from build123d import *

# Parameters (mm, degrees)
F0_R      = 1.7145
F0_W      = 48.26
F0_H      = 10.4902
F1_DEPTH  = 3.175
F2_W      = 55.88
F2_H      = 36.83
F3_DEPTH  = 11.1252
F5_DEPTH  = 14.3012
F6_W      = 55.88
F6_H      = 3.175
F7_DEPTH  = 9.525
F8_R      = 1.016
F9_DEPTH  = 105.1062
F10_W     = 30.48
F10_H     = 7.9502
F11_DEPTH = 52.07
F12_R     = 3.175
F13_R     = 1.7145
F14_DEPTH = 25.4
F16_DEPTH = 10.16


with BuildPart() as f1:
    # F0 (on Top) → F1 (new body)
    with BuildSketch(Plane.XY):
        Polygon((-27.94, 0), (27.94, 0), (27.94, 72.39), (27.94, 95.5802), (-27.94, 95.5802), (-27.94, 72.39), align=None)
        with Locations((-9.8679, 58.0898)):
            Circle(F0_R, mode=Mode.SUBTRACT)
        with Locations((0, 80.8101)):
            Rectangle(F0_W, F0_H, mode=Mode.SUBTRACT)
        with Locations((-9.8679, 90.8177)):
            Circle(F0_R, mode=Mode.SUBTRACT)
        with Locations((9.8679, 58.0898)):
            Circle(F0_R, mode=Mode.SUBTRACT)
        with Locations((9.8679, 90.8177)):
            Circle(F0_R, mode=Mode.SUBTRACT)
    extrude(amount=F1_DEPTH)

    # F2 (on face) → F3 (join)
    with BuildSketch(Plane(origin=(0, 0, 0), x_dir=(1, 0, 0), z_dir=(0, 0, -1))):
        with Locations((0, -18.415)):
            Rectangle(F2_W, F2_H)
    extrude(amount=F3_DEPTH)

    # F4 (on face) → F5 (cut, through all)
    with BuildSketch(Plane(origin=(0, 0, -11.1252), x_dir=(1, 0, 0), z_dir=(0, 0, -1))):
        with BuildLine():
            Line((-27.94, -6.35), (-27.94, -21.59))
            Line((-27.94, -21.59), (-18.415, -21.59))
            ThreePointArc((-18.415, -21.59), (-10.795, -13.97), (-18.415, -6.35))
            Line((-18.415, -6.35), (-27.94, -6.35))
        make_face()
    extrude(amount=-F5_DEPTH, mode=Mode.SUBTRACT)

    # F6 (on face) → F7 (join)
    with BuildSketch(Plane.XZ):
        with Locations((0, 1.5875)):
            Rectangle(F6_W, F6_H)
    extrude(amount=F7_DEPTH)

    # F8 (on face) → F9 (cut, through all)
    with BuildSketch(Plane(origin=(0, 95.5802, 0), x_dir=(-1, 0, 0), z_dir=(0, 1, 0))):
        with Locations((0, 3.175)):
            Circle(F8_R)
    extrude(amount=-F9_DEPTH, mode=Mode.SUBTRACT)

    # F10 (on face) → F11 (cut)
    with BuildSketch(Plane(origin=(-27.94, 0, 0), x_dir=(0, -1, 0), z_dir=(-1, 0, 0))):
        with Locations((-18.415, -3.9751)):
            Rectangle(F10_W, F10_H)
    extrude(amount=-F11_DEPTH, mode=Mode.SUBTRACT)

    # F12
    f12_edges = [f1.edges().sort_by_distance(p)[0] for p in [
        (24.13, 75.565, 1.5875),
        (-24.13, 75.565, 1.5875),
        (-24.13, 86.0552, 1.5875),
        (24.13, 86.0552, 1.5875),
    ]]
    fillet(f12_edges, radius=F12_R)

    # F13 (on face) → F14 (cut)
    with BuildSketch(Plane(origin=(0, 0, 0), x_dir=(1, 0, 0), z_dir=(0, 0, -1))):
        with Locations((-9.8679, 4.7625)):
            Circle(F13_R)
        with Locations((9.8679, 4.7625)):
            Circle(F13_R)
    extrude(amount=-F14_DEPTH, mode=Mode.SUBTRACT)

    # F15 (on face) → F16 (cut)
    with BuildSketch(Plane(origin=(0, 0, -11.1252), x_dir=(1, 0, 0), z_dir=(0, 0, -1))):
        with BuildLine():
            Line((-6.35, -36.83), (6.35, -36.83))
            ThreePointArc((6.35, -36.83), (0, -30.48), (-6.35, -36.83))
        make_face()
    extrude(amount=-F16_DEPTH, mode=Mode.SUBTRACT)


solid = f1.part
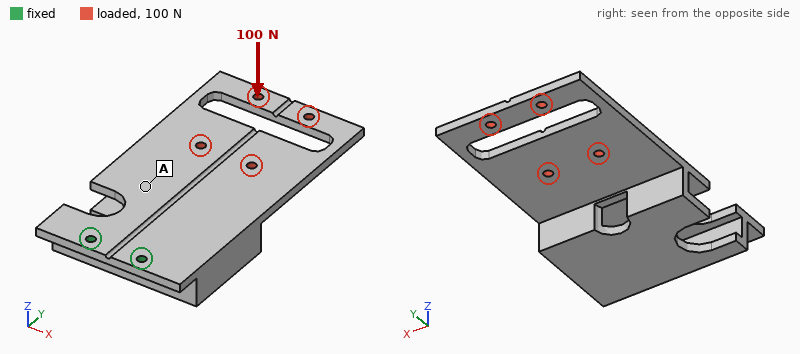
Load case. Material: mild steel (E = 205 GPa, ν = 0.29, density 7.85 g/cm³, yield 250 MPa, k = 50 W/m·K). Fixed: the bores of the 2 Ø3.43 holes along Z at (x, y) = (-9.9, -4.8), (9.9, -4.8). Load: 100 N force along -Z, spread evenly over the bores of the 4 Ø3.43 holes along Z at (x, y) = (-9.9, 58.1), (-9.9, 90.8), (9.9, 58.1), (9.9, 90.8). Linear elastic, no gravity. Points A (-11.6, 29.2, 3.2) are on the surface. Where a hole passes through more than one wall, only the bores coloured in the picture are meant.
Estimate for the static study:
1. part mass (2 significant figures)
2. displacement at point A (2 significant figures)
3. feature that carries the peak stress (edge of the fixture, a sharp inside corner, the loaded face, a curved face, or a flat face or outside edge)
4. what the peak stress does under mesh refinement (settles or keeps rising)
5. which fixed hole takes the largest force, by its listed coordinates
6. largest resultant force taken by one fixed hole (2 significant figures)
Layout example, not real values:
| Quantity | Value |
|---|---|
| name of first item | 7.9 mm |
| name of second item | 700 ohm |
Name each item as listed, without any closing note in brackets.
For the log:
| Quantity | Value |
|---|---|
| part mass | 200 g |
| displacement at point A | 0.084 mm |
| feature that carries the peak stress | edge of the fixture |
| what the peak stress does under mesh refinement | keeps rising |
| which fixed hole takes the largest force, by its listed coordinates | (9.9, -4.8) |
| largest resultant force taken by one fixed hole | 57 N |
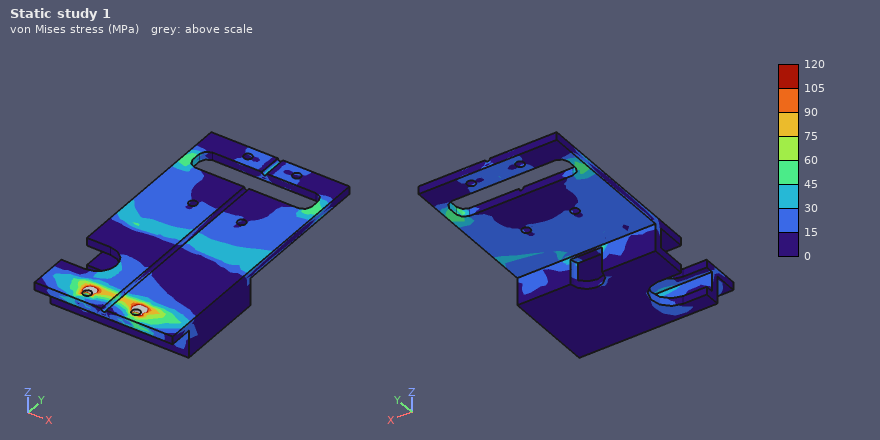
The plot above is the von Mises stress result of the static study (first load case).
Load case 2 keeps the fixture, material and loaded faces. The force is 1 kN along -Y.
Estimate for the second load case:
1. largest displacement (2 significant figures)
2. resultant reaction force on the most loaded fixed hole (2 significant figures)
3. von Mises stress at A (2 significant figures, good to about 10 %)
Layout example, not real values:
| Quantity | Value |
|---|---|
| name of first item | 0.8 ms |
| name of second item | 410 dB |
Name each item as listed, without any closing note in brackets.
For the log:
| Quantity | Value |
|---|---|
| largest displacement | 27 µm |
| resultant reaction force on the most loaded fixed hole | 510 N |
| von Mises stress at A | 11 MPa |
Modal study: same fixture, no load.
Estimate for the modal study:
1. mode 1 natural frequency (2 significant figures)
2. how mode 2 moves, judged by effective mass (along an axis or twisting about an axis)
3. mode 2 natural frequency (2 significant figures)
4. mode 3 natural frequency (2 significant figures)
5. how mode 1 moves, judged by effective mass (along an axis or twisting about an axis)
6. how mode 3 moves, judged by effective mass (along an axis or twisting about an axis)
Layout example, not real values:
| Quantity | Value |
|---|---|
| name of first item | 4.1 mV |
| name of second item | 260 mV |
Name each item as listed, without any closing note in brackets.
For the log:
| Quantity | Value |
|---|---|
| mode 1 natural frequency | 390 Hz |
| how mode 2 moves, judged by effective mass | along Z |
| mode 2 natural frequency | 1300 Hz |
| mode 3 natural frequency | 1700 Hz |
| how mode 1 moves, judged by effective mass | along Z |
| how mode 3 moves, judged by effective mass | twisting about Y |
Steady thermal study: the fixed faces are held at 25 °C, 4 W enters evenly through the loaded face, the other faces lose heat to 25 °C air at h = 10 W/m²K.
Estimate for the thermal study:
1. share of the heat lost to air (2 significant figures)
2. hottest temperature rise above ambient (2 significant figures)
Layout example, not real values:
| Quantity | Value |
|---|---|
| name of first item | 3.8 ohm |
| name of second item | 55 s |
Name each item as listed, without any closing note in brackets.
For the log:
| Quantity | Value |
|---|---|
| share of the heat lost to air | 49 % |
| hottest temperature rise above ambient | 45 K |
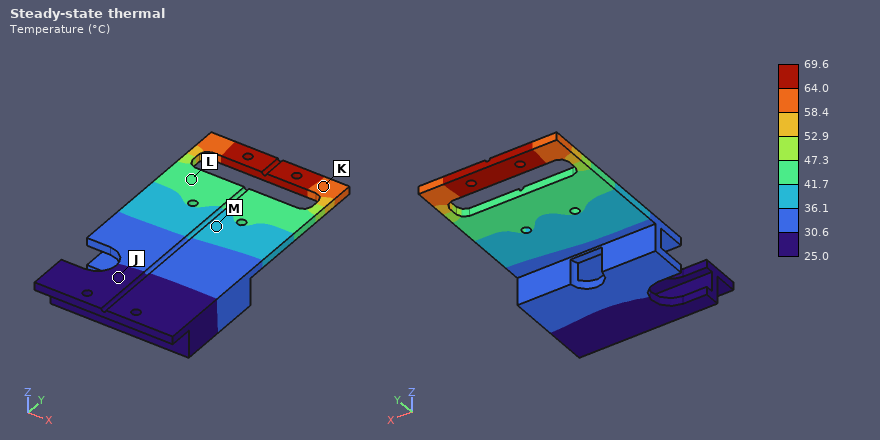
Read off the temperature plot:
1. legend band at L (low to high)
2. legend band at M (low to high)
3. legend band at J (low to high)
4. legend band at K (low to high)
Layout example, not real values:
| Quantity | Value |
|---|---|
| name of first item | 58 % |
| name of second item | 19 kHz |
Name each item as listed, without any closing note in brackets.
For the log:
| Quantity | Value |
|---|---|
| legend band at L | 41.7 to 47.3 °C |
| legend band at M | 36.1 to 41.7 °C |
| legend band at J | 25.0 to 30.6 °C |
| legend band at K | 58.4 to 64.0 °C |
